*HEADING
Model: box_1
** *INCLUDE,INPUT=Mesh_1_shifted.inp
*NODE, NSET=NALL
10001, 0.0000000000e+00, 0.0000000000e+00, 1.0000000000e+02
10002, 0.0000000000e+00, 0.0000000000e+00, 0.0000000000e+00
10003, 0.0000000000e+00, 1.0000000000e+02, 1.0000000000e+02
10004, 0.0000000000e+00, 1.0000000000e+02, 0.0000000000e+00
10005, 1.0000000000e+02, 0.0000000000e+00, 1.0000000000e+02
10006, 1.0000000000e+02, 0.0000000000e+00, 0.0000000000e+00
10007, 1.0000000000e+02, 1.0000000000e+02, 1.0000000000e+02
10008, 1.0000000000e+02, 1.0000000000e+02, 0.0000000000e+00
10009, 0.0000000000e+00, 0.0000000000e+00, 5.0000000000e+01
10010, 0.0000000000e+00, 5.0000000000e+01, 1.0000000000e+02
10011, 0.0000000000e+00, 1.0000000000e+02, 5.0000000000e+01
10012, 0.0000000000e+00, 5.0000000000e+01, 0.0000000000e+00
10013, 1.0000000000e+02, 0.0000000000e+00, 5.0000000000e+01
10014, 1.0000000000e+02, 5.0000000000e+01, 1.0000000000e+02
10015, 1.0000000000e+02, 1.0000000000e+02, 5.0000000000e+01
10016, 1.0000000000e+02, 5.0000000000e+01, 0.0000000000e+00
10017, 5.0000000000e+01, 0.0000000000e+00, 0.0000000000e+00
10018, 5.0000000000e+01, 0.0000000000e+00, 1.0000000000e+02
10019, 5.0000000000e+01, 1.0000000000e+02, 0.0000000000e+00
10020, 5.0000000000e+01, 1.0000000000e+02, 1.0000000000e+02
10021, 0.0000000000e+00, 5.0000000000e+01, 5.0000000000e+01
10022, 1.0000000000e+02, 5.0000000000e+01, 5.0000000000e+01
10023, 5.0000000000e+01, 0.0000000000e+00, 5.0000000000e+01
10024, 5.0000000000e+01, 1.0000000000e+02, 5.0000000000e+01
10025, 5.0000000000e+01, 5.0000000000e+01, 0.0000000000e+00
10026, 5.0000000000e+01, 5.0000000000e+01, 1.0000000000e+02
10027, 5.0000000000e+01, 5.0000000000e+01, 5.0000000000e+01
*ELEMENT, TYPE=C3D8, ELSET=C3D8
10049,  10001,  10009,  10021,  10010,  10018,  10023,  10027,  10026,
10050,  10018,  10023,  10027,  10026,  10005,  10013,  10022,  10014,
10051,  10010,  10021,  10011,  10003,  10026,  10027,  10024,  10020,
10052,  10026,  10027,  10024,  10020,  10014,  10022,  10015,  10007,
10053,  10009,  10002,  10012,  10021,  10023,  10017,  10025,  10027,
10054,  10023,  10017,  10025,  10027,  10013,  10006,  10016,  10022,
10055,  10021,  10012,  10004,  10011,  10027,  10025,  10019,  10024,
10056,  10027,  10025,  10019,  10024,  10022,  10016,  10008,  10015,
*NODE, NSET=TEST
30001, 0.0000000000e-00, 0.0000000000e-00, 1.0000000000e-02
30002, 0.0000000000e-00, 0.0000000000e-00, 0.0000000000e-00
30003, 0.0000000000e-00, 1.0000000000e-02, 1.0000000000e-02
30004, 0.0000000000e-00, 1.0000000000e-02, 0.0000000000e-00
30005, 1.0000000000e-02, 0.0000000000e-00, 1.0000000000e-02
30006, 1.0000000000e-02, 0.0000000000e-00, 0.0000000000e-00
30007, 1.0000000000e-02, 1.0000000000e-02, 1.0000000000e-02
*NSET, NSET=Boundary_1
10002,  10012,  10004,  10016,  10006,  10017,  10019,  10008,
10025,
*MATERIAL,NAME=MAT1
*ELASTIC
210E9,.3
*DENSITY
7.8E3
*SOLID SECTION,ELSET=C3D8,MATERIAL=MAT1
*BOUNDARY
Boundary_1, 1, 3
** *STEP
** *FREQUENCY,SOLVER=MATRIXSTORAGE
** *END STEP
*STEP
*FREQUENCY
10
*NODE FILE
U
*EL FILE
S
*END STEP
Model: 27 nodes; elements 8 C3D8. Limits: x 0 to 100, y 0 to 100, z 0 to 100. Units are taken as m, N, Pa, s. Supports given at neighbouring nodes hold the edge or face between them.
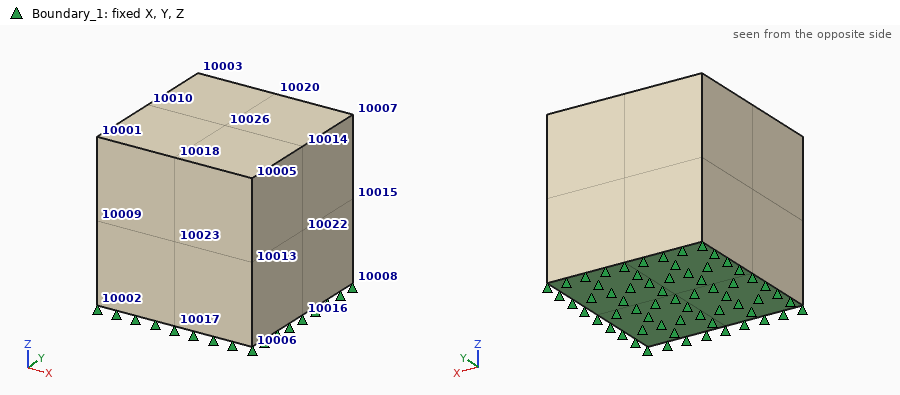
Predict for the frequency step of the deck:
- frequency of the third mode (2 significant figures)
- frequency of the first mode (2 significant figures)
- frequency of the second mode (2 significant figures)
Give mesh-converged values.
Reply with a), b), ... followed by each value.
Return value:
a) 7.5 Hz
b) 5.6 Hz
c) 5.6 Hz
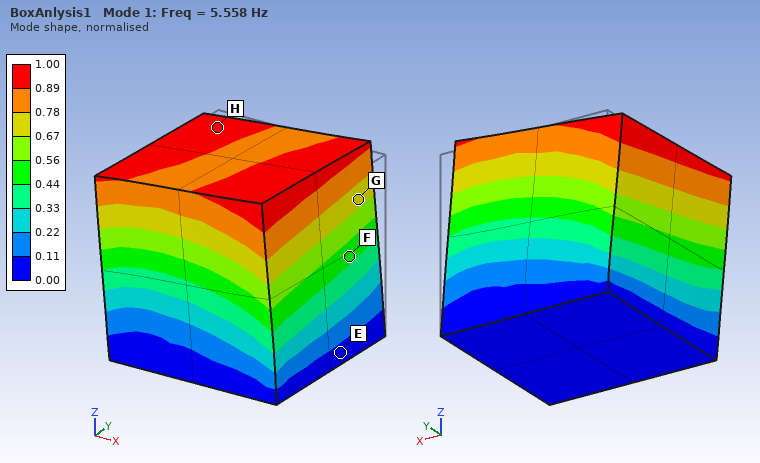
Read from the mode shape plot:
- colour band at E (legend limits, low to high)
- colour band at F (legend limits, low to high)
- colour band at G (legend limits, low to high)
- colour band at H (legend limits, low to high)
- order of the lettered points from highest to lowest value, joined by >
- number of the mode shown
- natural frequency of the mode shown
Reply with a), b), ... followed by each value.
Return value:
a) 0.00 to 0.11
b) 0.44 to 0.56
c) 0.67 to 0.78
d) 0.89 to 1.00
e) H > G > F > E
f) 1
g) 5.558 Hz
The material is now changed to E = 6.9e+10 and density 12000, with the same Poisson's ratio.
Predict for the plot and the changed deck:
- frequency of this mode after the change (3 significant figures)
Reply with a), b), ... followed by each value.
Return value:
a) 2.57 Hz
